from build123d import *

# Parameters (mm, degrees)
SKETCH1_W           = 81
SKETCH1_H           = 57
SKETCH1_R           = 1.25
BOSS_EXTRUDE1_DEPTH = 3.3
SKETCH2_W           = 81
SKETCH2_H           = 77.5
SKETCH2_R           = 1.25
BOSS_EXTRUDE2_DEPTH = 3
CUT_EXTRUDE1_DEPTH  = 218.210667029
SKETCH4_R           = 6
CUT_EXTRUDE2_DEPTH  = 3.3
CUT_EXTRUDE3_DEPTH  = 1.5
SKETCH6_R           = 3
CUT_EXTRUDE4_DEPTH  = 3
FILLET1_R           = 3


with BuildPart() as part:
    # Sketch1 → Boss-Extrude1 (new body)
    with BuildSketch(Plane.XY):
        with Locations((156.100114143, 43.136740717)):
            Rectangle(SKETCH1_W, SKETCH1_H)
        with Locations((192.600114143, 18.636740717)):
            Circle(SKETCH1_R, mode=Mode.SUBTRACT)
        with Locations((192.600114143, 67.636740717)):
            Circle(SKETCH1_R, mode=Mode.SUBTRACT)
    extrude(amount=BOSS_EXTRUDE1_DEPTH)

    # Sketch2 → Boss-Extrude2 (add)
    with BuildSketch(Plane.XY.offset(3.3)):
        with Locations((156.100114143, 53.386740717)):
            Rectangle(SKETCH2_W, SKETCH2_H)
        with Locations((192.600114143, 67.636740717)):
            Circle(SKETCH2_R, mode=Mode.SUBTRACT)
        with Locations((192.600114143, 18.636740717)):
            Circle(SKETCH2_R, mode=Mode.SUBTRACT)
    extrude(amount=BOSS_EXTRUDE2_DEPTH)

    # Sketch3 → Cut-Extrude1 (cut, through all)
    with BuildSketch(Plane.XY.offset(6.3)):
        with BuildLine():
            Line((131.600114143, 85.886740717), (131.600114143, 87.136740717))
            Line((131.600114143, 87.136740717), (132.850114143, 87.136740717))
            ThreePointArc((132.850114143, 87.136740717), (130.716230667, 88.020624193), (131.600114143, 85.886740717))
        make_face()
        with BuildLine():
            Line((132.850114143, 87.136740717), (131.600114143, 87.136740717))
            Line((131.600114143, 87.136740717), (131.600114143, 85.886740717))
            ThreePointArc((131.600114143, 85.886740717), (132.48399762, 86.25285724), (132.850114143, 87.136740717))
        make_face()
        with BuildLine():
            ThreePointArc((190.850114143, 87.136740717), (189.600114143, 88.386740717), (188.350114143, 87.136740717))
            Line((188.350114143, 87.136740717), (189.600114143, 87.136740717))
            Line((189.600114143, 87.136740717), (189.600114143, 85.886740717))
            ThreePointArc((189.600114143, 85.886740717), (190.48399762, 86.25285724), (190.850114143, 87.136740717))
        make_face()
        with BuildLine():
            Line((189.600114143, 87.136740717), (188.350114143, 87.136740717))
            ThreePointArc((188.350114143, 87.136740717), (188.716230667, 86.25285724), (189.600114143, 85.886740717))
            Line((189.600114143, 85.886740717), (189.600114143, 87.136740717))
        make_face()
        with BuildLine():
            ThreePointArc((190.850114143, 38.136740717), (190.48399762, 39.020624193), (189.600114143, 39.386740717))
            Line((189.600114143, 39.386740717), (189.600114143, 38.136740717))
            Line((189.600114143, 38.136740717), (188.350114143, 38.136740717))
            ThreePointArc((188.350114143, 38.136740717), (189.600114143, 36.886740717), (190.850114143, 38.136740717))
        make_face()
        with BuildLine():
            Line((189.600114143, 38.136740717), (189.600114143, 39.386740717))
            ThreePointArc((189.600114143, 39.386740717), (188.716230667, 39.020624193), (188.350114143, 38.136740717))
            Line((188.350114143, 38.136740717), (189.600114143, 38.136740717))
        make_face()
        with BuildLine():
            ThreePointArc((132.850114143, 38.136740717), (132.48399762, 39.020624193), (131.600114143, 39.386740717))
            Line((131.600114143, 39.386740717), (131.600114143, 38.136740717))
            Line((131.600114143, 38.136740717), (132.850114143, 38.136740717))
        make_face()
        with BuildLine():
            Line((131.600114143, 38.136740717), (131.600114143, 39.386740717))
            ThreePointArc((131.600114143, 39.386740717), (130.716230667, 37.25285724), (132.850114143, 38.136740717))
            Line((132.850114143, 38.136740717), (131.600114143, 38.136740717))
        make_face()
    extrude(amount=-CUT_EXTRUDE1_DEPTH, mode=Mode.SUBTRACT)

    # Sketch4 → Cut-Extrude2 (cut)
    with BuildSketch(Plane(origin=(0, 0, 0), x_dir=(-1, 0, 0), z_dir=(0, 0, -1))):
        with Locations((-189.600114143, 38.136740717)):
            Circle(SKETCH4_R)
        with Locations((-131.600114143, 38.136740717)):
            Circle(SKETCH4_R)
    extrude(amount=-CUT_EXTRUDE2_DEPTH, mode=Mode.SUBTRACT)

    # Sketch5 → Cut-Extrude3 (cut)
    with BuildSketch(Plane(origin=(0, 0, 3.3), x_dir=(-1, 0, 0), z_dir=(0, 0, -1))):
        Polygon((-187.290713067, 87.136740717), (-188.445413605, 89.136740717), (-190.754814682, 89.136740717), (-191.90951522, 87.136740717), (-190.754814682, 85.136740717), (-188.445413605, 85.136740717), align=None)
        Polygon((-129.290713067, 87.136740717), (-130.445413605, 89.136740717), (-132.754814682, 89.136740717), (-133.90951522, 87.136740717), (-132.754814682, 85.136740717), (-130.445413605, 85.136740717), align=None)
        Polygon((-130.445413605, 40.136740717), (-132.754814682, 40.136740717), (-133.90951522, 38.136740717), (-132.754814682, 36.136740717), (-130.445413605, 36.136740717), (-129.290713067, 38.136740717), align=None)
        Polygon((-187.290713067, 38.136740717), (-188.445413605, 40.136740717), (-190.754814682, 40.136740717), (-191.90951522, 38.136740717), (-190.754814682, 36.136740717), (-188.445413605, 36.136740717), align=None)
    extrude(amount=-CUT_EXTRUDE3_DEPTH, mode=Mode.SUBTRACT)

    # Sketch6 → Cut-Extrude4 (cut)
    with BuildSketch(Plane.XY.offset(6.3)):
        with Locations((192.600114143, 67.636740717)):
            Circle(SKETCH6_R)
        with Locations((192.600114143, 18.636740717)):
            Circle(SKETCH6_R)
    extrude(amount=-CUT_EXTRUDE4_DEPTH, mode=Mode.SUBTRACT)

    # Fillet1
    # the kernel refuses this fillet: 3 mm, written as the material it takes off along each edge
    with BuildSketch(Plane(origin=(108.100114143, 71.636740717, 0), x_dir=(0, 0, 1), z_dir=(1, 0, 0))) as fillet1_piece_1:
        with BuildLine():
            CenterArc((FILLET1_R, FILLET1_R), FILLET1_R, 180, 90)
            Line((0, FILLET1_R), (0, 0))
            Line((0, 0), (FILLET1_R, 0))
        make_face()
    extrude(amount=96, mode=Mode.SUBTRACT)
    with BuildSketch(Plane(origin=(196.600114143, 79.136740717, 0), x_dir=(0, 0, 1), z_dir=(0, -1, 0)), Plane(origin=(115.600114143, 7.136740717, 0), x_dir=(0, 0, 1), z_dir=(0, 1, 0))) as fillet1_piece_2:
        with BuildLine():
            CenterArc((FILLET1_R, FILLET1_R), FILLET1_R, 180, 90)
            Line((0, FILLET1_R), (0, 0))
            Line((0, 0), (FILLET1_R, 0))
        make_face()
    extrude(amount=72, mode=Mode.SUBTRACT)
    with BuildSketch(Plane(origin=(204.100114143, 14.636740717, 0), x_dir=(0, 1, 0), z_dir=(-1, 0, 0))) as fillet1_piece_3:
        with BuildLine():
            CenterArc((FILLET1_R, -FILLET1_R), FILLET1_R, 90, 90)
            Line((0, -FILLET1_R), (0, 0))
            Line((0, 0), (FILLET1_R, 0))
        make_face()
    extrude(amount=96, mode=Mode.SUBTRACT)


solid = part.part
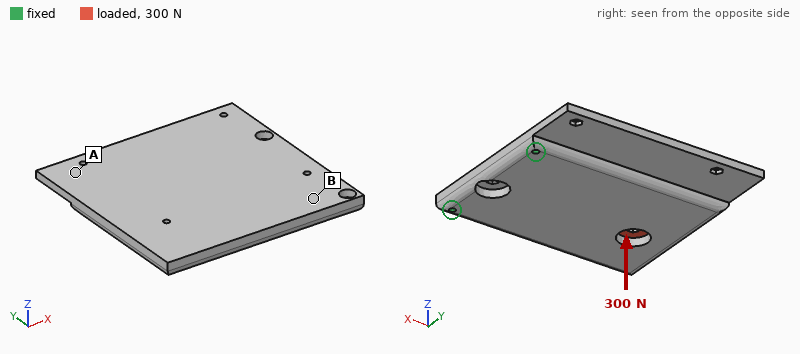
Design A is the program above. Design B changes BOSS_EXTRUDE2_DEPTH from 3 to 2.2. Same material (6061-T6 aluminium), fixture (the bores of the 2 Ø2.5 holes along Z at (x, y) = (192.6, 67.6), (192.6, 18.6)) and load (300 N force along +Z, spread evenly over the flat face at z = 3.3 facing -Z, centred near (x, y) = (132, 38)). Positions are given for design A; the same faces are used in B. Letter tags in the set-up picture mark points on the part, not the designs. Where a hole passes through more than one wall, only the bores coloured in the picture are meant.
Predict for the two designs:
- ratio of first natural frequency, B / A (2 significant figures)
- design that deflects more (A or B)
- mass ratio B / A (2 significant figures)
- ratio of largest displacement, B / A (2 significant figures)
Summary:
0.98
B
0.85
1.3
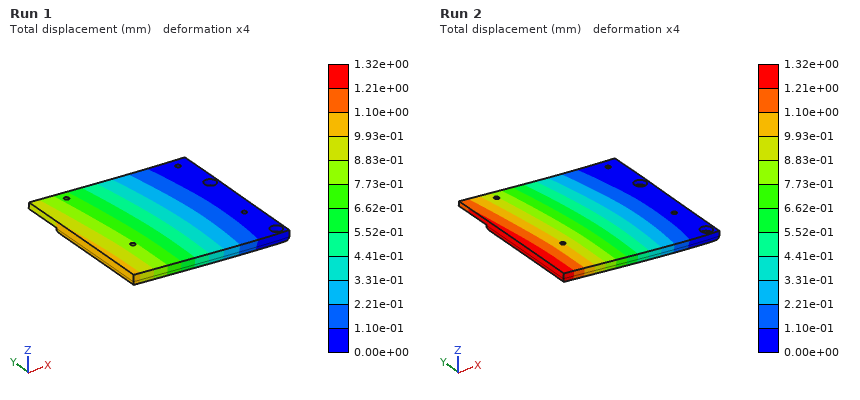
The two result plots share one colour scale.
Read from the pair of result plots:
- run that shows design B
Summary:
Run 2
